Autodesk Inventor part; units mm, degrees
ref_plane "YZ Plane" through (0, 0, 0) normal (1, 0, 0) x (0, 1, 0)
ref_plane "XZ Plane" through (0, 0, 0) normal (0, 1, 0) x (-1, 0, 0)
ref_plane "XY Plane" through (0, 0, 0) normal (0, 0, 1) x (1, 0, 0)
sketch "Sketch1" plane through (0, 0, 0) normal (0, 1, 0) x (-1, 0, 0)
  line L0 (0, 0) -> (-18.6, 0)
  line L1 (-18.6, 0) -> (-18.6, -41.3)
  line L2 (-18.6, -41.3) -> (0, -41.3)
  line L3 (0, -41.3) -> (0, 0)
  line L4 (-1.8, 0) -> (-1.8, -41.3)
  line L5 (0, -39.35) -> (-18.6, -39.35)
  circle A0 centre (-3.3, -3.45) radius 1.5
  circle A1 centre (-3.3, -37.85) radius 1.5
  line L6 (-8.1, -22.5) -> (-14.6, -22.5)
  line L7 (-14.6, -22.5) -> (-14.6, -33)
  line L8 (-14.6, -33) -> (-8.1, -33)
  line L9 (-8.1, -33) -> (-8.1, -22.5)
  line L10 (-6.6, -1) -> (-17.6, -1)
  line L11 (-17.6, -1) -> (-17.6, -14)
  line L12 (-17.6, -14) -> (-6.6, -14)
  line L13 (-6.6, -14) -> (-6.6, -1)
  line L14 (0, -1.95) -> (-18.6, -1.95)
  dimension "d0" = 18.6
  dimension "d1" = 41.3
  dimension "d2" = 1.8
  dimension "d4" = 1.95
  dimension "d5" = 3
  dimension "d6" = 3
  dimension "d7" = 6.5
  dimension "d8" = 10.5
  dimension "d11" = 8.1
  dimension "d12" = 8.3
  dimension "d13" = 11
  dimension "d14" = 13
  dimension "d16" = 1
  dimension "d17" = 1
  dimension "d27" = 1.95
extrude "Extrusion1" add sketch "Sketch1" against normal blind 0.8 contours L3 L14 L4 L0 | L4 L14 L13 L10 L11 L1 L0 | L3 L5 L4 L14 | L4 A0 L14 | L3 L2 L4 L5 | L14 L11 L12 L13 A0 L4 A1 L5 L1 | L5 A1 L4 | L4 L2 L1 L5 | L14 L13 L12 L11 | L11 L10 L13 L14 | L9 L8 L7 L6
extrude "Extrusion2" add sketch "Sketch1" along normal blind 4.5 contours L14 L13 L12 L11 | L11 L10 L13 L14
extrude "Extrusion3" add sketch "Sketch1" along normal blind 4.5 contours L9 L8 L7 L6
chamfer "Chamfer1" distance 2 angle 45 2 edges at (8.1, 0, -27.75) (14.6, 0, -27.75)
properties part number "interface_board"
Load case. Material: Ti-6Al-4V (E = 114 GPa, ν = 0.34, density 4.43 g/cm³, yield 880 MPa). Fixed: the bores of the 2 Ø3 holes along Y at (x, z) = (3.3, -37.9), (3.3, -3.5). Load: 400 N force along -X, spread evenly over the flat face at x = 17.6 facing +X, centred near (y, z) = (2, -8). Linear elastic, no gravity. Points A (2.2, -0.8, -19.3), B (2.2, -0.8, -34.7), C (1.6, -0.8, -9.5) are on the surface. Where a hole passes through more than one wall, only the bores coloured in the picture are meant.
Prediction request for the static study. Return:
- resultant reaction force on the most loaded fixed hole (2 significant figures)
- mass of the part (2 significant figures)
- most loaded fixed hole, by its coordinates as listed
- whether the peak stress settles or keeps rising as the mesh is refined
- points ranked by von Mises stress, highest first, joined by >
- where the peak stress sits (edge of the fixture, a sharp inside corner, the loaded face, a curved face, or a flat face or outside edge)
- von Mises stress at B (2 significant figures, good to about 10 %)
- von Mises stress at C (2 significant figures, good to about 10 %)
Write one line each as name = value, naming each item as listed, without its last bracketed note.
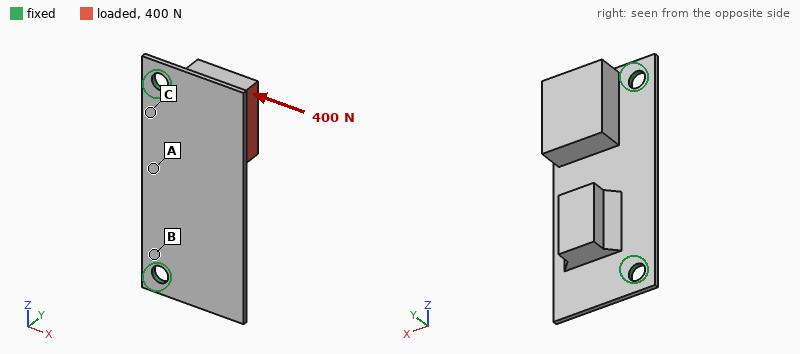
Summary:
resultant reaction force on the most loaded fixed hole = 360 N
mass of the part = 7.1 g
most loaded fixed hole, by its coordinates as listed = (3.3, -3.5)
whether the peak stress settles or keeps rising as the mesh is refined = keeps rising
points ranked by von Mises stress, highest first, joined by > = C > B > A
where the peak stress sits = edge of the fixture
von Mises stress at B = 110 MPa
von Mises stress at C = 170 MPa
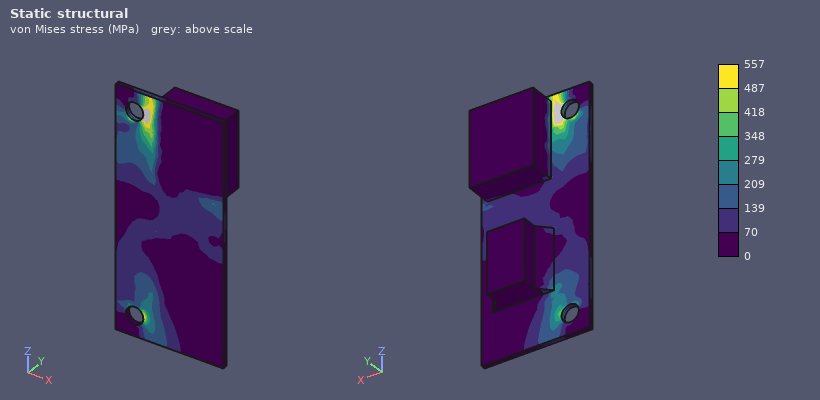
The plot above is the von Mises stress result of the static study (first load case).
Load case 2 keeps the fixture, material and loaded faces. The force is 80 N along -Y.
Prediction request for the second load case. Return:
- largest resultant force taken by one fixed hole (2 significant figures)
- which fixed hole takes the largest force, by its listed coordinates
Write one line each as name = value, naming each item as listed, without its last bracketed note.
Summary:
largest resultant force taken by one fixed hole = 73 N
which fixed hole takes the largest force, by its listed coordinates = (3.3, -3.5)
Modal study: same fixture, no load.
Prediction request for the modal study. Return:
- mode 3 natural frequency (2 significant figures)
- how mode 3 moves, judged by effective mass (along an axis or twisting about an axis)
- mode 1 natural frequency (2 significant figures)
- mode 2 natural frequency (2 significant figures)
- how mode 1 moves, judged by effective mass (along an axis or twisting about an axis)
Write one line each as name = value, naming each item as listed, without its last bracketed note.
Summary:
mode 3 natural frequency = 4100 Hz
how mode 3 moves, judged by effective mass = twisting about X
mode 1 natural frequency = 1400 Hz
mode 2 natural frequency = 3700 Hz
how mode 1 moves, judged by effective mass = along Y
